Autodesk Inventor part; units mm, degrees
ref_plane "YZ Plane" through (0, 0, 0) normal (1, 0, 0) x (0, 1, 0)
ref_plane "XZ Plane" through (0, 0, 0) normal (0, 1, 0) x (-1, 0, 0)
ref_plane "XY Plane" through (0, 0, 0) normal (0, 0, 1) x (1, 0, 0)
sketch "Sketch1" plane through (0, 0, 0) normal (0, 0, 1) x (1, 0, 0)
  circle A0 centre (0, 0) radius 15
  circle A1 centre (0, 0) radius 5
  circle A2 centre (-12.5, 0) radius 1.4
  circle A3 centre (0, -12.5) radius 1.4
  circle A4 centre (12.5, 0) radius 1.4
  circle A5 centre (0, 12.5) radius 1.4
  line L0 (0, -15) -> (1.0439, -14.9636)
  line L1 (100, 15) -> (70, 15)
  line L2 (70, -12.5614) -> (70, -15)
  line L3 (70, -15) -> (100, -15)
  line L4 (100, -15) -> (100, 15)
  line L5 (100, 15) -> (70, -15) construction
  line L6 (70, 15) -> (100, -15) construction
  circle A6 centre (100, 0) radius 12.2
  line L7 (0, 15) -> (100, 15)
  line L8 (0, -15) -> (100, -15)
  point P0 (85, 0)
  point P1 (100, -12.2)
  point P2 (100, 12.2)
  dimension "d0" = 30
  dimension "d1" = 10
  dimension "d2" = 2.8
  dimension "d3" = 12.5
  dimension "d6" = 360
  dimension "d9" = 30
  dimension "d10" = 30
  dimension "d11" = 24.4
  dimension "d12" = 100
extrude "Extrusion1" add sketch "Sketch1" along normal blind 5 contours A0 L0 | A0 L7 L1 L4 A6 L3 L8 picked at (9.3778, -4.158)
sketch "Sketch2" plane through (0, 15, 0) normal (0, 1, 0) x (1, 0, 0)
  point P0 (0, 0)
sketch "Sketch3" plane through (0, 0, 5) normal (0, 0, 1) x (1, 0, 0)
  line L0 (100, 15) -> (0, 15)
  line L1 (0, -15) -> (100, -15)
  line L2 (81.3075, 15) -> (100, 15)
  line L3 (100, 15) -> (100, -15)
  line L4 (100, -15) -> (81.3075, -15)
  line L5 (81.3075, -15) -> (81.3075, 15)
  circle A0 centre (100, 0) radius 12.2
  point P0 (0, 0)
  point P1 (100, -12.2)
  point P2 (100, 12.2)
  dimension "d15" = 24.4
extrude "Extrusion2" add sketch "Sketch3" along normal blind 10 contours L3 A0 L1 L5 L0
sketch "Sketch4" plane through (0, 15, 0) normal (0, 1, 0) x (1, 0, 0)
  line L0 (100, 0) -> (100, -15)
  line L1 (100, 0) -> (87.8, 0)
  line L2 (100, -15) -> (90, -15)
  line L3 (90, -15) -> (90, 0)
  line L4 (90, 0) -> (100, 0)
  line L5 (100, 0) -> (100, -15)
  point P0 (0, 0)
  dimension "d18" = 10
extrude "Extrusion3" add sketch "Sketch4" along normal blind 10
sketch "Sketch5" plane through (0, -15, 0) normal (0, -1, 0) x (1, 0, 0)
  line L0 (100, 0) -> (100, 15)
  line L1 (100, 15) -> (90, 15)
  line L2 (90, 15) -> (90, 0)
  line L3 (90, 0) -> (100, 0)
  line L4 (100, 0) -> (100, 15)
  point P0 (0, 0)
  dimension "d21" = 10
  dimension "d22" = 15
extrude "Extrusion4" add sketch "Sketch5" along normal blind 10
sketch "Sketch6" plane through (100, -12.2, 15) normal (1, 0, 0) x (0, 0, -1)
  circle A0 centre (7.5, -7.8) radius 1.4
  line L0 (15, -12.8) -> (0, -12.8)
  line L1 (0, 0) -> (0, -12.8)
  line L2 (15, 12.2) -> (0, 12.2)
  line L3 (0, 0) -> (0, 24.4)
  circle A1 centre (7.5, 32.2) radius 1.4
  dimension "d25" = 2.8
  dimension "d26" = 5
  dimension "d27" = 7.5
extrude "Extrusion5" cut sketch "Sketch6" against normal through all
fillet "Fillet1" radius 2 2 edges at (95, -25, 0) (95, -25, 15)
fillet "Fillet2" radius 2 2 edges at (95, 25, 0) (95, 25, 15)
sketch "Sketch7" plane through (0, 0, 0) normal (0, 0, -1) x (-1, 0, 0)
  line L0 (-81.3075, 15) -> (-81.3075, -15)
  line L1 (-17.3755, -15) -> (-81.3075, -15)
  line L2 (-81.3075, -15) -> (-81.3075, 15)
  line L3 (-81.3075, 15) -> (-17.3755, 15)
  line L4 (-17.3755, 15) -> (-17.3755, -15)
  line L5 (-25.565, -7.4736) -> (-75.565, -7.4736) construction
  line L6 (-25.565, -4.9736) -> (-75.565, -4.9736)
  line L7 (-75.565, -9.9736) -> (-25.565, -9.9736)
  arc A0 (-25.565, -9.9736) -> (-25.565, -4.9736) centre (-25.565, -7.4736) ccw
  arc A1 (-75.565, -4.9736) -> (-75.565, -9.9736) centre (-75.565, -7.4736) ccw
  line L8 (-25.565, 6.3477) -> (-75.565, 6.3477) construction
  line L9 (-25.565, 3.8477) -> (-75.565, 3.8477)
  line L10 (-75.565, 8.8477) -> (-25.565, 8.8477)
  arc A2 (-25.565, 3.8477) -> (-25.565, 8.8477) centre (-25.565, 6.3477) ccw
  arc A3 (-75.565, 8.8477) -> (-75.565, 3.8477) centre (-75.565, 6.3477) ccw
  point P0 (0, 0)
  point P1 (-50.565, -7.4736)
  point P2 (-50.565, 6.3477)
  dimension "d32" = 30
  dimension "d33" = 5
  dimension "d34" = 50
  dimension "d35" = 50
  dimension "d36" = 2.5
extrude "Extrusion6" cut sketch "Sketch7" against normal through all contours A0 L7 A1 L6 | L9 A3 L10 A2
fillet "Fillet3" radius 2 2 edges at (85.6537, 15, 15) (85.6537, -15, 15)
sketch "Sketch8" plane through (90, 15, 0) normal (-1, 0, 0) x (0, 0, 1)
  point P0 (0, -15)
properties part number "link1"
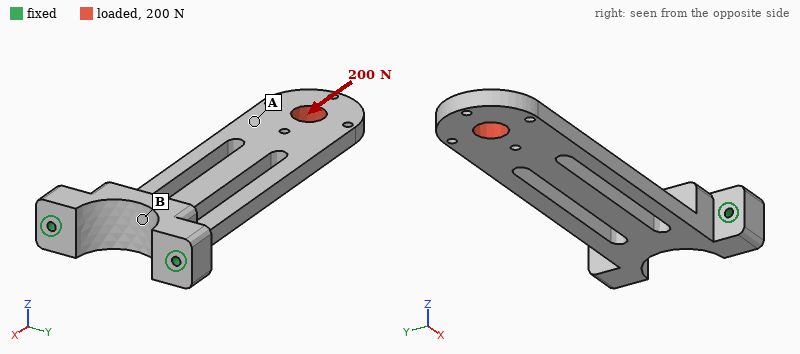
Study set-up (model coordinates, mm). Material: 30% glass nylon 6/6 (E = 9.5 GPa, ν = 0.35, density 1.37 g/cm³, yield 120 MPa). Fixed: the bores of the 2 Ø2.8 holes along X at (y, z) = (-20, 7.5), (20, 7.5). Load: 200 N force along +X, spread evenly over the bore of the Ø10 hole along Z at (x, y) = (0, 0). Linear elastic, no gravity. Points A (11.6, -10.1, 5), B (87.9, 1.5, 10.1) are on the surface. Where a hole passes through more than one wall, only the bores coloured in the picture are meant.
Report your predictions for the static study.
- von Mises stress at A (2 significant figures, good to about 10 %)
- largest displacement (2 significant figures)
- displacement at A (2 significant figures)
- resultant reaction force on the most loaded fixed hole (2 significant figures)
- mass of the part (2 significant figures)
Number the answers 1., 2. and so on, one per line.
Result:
1. 1.4 MPa
2. 92 µm
3. 69 µm
4. 120 N
5. 25 g
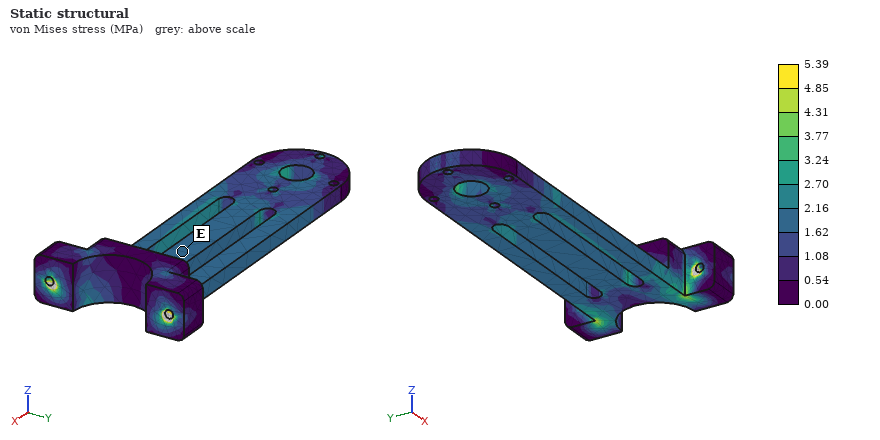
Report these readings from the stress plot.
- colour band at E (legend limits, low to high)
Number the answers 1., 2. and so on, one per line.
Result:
1. 1.62 to 2.16 MPa
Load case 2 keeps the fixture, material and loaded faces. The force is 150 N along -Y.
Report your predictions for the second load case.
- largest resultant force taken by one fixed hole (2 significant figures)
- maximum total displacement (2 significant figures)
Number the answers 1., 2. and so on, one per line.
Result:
1. 480 N
2. 1.3 mm
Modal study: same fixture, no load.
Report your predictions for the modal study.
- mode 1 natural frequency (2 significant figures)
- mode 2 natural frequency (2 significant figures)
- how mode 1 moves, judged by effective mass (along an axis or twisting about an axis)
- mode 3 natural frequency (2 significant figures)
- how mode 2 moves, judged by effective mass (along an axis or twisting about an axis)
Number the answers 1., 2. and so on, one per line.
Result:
1. 200 Hz
2. 660 Hz
3. along Z
4. 1100 Hz
5. along Y
